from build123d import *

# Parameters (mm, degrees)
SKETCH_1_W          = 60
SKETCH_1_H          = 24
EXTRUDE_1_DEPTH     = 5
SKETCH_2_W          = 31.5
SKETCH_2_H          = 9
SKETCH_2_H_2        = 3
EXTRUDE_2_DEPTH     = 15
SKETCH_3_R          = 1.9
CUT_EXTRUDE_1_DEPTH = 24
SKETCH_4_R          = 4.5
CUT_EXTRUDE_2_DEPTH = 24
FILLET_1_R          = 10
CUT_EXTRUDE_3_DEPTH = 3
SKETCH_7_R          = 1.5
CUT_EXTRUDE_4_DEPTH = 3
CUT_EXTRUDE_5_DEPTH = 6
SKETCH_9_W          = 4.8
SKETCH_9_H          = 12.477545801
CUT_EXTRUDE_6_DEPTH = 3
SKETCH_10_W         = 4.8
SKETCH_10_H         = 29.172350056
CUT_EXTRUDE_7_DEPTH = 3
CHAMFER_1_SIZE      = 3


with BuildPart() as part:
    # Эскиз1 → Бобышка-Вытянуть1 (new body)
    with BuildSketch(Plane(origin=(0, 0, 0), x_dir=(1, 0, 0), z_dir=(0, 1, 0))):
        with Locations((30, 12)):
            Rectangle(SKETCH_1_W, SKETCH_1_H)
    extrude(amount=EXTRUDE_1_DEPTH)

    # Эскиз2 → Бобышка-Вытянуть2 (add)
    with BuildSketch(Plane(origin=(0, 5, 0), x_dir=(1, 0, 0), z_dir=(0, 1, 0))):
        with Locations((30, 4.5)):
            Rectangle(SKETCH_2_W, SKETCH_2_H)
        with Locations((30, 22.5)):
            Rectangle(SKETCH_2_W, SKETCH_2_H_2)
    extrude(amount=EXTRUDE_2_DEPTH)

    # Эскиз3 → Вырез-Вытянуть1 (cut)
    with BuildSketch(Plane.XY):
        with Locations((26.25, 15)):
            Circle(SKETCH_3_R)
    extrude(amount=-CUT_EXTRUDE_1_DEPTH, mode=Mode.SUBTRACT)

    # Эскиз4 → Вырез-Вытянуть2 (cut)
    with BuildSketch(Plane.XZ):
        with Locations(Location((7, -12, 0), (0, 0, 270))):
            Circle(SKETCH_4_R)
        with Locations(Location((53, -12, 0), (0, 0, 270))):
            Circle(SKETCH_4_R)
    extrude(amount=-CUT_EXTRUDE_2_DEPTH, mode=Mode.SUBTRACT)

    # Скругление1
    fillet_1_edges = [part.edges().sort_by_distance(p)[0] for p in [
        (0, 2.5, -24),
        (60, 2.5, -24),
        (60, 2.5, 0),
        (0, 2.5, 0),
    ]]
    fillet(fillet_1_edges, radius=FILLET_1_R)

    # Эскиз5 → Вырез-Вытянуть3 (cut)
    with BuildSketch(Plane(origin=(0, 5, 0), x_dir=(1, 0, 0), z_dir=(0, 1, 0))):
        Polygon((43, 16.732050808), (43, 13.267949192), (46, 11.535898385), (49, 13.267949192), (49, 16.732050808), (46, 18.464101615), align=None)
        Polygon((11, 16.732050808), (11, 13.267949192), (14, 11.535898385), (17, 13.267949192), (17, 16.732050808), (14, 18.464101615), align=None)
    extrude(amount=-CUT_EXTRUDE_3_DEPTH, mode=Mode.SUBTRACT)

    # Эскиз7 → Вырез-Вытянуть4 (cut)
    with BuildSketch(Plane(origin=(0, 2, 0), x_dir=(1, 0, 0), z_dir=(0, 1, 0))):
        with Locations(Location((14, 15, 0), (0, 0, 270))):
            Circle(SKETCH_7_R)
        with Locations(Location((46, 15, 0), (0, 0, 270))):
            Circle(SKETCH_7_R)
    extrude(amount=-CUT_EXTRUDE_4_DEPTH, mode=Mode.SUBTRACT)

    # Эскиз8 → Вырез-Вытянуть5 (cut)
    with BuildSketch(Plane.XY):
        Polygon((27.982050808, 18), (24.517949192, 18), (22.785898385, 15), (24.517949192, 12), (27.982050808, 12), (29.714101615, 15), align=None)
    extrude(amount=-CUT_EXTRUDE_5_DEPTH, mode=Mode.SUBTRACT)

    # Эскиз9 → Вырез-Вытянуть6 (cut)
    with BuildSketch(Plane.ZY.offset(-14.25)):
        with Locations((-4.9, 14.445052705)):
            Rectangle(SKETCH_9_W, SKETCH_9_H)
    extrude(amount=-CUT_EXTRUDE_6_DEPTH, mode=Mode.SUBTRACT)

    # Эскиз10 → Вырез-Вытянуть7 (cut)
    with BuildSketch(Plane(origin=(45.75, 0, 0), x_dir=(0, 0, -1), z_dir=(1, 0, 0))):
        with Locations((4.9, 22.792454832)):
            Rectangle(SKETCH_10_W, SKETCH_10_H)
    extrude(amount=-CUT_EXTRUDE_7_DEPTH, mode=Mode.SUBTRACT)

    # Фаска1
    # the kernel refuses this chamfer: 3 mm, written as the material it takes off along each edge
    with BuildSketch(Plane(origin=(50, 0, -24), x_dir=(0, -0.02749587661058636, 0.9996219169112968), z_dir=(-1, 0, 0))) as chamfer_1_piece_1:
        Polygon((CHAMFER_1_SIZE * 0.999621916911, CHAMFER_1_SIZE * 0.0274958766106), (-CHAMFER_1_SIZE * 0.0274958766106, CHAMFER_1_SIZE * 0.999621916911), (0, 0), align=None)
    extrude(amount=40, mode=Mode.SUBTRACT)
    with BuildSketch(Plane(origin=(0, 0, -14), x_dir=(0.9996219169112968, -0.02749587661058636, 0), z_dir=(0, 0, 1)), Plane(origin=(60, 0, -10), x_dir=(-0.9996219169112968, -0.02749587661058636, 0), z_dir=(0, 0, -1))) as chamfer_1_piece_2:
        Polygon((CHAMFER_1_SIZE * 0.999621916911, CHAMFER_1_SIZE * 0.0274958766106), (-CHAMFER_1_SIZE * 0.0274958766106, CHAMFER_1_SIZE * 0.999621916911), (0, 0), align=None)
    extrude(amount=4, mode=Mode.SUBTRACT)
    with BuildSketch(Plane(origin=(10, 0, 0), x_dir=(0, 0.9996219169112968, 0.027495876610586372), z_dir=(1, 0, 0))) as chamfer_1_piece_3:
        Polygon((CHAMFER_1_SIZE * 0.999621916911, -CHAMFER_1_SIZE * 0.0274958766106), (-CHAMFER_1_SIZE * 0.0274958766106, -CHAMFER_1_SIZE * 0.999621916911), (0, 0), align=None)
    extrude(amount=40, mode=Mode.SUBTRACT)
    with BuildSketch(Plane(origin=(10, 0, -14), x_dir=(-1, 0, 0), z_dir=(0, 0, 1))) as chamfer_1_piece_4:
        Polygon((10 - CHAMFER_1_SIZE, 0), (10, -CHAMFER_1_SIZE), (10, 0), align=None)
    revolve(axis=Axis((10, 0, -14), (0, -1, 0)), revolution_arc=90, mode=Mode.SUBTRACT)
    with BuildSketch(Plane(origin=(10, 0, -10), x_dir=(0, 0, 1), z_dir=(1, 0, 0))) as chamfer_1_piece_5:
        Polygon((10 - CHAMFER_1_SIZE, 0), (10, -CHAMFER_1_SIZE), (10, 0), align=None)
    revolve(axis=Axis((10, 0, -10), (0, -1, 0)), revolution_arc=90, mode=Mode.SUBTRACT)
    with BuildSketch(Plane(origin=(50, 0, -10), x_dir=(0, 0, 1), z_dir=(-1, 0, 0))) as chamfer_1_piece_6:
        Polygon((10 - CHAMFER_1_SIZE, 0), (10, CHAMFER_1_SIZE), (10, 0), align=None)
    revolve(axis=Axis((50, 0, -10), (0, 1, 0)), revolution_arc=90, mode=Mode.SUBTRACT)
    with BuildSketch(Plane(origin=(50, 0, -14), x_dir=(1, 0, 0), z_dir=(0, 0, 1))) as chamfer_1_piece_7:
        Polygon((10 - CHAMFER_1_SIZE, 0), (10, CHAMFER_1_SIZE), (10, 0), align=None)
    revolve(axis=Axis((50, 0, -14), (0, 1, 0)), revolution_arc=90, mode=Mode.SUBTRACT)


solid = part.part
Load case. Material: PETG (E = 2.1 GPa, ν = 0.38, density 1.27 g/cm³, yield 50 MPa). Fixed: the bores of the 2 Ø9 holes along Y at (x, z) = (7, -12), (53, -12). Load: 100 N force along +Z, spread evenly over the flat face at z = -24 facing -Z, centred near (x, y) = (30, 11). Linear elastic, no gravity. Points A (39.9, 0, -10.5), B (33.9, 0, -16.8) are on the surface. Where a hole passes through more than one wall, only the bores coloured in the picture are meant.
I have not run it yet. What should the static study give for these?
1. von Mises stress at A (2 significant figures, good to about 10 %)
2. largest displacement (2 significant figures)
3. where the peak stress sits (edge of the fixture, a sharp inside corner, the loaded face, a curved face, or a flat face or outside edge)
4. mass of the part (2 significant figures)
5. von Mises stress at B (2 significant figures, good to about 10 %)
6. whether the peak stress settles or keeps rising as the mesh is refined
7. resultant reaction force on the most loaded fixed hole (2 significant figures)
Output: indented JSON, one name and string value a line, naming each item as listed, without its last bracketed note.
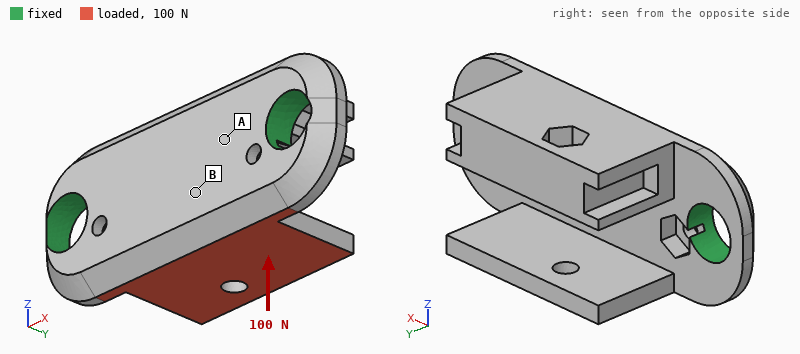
{
  "von Mises stress at A": "1.3 MPa",
  "largest displacement": "0.55 mm",
  "where the peak stress sits": "a sharp inside corner",
  "mass of the part": "13 g",
  "von Mises stress at B": "3.6 MPa",
  "whether the peak stress settles or keeps rising as the mesh is refined": "keeps rising",
  "resultant reaction force on the most loaded fixed hole": "50 N"
}
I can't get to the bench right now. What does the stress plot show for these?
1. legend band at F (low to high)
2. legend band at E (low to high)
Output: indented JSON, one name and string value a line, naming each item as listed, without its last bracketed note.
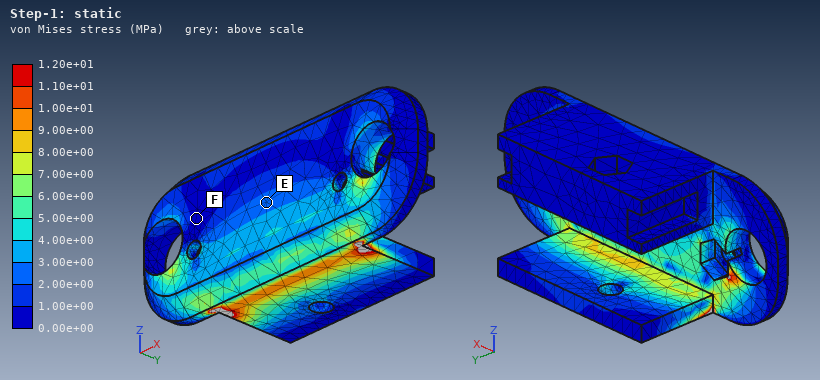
{
  "legend band at F": "0.00e+00 to 1.00e+00 MPa",
  "legend band at E": "2.00e+00 to 3.00e+00 MPa"
}
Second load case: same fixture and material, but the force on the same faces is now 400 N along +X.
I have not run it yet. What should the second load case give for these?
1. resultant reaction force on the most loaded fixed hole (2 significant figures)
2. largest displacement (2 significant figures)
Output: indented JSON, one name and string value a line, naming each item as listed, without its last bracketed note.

{
  "resultant reaction force on the most loaded fixed hole": "240 N",
  "largest displacement": "0.23 mm"
}
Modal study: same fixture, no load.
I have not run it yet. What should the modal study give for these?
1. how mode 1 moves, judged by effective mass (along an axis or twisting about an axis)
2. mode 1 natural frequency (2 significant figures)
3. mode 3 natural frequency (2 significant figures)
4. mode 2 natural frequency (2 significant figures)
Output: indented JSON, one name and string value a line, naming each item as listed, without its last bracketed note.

{
  "how mode 1 moves, judged by effective mass": "along Z",
  "mode 1 natural frequency": "1700 Hz",
  "mode 3 natural frequency": "3000 Hz",
  "mode 2 natural frequency": "2200 Hz"
}
